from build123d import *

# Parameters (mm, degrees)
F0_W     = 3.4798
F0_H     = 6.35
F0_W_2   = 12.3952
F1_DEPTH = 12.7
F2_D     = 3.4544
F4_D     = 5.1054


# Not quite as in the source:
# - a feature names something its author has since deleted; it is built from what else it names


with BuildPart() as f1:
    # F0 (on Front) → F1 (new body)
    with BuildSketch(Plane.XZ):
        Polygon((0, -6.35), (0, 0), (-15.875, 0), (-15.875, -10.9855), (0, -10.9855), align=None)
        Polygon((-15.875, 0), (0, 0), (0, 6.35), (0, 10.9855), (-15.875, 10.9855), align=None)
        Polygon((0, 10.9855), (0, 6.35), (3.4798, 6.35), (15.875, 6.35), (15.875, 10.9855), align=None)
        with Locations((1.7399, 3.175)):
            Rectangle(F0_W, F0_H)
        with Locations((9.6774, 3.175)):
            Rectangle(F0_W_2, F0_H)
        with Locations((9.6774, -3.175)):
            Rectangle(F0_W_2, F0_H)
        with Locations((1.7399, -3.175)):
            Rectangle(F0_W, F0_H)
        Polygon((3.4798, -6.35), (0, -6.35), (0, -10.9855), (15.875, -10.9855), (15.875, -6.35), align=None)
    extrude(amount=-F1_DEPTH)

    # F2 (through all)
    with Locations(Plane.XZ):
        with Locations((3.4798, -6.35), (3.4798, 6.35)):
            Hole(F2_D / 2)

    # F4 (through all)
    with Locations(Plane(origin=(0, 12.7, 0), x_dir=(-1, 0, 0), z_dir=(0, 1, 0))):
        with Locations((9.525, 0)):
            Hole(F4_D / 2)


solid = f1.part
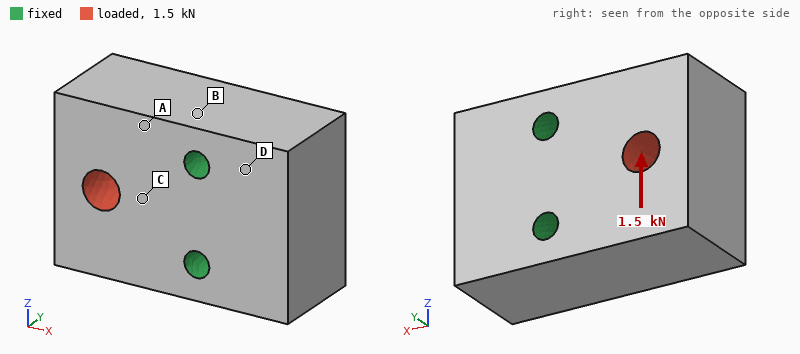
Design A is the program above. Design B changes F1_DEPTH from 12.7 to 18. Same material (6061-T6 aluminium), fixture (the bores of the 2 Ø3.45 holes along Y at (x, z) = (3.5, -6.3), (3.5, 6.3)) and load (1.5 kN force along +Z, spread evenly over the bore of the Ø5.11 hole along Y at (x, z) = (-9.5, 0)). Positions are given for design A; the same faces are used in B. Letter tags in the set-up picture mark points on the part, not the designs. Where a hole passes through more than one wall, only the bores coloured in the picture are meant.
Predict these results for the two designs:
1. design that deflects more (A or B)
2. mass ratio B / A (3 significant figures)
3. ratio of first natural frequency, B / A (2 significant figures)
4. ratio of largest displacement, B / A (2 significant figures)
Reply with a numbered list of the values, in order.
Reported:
1. A
2. 1.42
3. 1.2
4. 0.70
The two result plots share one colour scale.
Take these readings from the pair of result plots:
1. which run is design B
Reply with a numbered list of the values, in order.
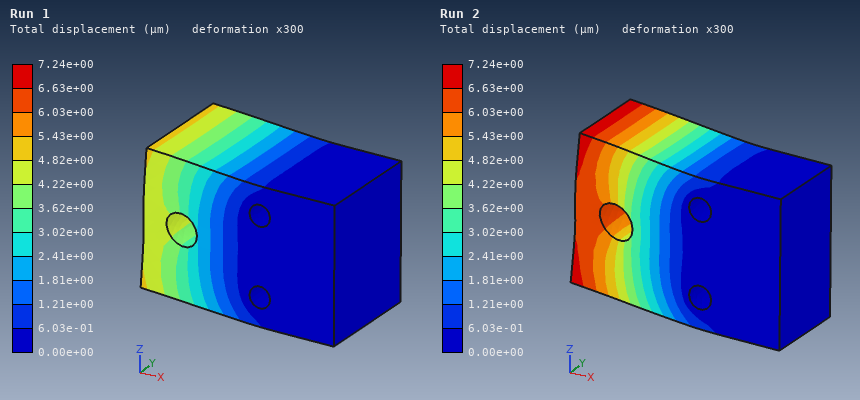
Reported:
1. Run 1
